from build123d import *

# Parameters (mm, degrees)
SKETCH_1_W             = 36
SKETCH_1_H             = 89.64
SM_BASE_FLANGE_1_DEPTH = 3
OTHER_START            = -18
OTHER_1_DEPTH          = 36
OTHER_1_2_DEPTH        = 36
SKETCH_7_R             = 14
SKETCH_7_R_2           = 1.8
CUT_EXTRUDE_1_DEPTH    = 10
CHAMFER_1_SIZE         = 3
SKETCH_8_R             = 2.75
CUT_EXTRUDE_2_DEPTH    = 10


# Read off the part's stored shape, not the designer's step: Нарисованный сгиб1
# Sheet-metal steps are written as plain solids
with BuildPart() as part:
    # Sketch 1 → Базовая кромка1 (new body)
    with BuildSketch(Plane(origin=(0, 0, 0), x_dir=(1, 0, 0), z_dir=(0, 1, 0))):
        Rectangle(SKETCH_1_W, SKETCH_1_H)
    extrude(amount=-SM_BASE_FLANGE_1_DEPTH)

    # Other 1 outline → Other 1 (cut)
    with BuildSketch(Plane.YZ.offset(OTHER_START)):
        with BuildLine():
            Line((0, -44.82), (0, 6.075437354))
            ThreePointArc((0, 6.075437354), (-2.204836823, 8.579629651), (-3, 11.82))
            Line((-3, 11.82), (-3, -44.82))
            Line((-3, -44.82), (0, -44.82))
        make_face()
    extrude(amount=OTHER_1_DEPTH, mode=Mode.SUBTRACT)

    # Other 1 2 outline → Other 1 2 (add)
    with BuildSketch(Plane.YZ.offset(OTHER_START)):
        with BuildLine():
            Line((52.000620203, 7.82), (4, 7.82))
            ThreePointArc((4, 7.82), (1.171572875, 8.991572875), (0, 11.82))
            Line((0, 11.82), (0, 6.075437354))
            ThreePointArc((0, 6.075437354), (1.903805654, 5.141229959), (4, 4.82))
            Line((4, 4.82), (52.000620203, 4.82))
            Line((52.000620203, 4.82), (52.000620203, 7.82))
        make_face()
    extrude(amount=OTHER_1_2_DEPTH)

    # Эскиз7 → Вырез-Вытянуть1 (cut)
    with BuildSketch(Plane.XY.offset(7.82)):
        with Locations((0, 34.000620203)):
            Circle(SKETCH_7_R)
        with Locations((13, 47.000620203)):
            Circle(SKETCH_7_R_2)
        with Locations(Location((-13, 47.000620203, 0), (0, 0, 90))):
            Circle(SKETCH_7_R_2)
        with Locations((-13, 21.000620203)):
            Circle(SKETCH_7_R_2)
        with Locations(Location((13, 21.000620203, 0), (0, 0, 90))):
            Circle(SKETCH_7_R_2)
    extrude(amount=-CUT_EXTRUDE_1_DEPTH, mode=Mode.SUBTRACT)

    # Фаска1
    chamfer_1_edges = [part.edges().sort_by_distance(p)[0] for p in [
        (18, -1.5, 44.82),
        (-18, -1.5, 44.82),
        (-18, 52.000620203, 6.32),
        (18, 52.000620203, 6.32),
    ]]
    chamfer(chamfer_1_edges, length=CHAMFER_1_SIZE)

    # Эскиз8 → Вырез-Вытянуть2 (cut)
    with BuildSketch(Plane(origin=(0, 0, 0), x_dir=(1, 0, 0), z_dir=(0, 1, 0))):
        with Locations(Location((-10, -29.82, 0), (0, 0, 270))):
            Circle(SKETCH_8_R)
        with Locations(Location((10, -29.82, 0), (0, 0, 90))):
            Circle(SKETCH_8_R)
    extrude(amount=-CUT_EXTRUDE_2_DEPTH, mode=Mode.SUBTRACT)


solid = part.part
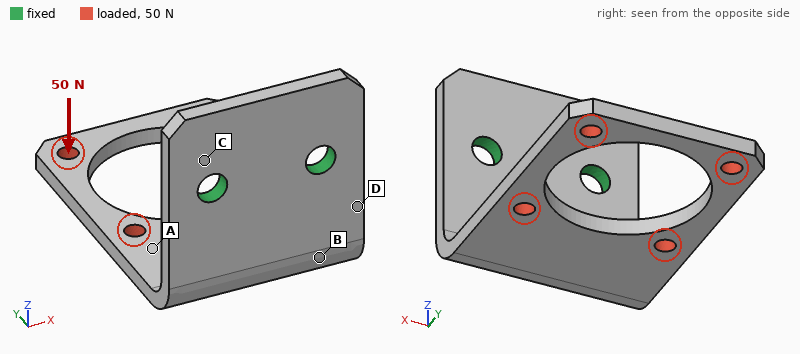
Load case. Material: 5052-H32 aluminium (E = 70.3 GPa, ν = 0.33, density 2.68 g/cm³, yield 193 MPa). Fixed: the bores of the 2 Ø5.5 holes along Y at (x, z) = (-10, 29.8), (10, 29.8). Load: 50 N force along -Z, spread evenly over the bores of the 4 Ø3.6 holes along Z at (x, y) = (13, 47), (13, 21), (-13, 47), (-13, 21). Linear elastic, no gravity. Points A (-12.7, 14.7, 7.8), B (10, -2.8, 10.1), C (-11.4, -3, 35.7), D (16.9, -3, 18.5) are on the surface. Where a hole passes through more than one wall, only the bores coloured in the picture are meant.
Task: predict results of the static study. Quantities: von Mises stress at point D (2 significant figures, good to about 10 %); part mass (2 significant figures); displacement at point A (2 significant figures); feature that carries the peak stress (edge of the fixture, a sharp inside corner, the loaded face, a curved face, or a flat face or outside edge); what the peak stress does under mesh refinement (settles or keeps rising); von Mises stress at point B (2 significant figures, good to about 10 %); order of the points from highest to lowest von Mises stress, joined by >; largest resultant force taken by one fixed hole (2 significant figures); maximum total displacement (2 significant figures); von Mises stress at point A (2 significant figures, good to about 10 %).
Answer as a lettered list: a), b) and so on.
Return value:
a) 34 MPa
b) 20 g
c) 0.14 mm
d) edge of the fixture
e) keeps rising
f) 25 MPa
g) D > B > A > C
h) 28 N
i) 0.65 mm
j) 20 MPa
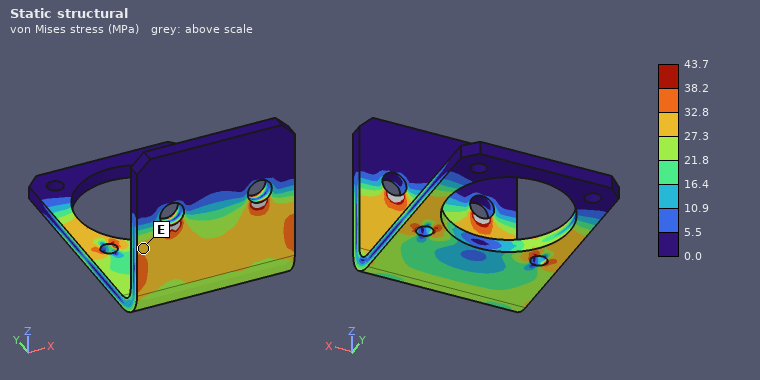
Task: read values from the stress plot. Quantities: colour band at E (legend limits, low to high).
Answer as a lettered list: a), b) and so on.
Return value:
a) 27.3 to 32.8 MPa
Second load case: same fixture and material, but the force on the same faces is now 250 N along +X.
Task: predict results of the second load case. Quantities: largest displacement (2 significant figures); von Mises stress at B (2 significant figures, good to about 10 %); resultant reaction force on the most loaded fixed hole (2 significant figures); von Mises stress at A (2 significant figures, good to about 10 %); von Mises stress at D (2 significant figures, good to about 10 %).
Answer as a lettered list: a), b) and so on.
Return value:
a) 0.69 mm
b) 74 MPa
c) 450 N
d) 20 MPa
e) 68 MPa
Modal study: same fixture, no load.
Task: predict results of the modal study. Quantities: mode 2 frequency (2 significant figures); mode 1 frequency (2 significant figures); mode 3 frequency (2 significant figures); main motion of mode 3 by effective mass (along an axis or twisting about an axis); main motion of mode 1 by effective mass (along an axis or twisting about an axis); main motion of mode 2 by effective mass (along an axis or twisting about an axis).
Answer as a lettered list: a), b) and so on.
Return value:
a) 1400 Hz
b) 710 Hz
c) 2300 Hz
d) along Y
e) along Z
f) along X
